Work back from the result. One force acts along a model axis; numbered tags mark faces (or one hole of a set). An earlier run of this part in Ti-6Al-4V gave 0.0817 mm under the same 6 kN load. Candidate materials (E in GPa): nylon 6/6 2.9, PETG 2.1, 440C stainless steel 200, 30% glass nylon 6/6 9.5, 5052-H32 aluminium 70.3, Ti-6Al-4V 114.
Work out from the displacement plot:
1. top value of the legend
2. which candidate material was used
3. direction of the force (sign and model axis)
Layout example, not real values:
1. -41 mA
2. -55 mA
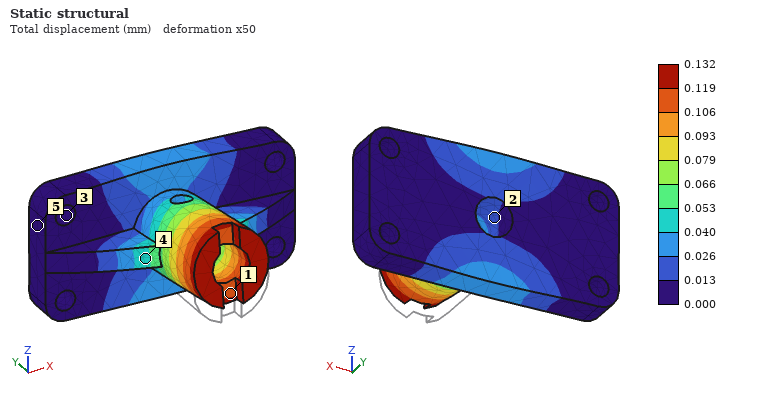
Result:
1. 0.132 mm
2. 5052-H32 aluminium
3. +Z
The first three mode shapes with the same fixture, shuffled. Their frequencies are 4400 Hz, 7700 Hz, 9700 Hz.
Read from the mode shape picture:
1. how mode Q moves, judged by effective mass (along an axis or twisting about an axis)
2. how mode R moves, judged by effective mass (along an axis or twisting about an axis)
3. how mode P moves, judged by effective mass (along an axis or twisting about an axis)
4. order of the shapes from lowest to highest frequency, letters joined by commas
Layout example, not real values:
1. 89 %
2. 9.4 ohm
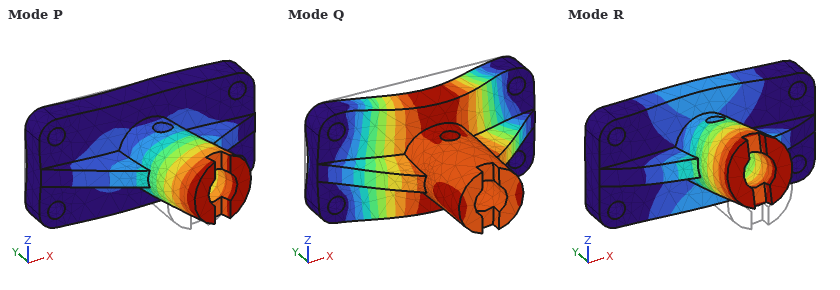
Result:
1. along Y
2. along Z
3. along X
4. R, Q, P
